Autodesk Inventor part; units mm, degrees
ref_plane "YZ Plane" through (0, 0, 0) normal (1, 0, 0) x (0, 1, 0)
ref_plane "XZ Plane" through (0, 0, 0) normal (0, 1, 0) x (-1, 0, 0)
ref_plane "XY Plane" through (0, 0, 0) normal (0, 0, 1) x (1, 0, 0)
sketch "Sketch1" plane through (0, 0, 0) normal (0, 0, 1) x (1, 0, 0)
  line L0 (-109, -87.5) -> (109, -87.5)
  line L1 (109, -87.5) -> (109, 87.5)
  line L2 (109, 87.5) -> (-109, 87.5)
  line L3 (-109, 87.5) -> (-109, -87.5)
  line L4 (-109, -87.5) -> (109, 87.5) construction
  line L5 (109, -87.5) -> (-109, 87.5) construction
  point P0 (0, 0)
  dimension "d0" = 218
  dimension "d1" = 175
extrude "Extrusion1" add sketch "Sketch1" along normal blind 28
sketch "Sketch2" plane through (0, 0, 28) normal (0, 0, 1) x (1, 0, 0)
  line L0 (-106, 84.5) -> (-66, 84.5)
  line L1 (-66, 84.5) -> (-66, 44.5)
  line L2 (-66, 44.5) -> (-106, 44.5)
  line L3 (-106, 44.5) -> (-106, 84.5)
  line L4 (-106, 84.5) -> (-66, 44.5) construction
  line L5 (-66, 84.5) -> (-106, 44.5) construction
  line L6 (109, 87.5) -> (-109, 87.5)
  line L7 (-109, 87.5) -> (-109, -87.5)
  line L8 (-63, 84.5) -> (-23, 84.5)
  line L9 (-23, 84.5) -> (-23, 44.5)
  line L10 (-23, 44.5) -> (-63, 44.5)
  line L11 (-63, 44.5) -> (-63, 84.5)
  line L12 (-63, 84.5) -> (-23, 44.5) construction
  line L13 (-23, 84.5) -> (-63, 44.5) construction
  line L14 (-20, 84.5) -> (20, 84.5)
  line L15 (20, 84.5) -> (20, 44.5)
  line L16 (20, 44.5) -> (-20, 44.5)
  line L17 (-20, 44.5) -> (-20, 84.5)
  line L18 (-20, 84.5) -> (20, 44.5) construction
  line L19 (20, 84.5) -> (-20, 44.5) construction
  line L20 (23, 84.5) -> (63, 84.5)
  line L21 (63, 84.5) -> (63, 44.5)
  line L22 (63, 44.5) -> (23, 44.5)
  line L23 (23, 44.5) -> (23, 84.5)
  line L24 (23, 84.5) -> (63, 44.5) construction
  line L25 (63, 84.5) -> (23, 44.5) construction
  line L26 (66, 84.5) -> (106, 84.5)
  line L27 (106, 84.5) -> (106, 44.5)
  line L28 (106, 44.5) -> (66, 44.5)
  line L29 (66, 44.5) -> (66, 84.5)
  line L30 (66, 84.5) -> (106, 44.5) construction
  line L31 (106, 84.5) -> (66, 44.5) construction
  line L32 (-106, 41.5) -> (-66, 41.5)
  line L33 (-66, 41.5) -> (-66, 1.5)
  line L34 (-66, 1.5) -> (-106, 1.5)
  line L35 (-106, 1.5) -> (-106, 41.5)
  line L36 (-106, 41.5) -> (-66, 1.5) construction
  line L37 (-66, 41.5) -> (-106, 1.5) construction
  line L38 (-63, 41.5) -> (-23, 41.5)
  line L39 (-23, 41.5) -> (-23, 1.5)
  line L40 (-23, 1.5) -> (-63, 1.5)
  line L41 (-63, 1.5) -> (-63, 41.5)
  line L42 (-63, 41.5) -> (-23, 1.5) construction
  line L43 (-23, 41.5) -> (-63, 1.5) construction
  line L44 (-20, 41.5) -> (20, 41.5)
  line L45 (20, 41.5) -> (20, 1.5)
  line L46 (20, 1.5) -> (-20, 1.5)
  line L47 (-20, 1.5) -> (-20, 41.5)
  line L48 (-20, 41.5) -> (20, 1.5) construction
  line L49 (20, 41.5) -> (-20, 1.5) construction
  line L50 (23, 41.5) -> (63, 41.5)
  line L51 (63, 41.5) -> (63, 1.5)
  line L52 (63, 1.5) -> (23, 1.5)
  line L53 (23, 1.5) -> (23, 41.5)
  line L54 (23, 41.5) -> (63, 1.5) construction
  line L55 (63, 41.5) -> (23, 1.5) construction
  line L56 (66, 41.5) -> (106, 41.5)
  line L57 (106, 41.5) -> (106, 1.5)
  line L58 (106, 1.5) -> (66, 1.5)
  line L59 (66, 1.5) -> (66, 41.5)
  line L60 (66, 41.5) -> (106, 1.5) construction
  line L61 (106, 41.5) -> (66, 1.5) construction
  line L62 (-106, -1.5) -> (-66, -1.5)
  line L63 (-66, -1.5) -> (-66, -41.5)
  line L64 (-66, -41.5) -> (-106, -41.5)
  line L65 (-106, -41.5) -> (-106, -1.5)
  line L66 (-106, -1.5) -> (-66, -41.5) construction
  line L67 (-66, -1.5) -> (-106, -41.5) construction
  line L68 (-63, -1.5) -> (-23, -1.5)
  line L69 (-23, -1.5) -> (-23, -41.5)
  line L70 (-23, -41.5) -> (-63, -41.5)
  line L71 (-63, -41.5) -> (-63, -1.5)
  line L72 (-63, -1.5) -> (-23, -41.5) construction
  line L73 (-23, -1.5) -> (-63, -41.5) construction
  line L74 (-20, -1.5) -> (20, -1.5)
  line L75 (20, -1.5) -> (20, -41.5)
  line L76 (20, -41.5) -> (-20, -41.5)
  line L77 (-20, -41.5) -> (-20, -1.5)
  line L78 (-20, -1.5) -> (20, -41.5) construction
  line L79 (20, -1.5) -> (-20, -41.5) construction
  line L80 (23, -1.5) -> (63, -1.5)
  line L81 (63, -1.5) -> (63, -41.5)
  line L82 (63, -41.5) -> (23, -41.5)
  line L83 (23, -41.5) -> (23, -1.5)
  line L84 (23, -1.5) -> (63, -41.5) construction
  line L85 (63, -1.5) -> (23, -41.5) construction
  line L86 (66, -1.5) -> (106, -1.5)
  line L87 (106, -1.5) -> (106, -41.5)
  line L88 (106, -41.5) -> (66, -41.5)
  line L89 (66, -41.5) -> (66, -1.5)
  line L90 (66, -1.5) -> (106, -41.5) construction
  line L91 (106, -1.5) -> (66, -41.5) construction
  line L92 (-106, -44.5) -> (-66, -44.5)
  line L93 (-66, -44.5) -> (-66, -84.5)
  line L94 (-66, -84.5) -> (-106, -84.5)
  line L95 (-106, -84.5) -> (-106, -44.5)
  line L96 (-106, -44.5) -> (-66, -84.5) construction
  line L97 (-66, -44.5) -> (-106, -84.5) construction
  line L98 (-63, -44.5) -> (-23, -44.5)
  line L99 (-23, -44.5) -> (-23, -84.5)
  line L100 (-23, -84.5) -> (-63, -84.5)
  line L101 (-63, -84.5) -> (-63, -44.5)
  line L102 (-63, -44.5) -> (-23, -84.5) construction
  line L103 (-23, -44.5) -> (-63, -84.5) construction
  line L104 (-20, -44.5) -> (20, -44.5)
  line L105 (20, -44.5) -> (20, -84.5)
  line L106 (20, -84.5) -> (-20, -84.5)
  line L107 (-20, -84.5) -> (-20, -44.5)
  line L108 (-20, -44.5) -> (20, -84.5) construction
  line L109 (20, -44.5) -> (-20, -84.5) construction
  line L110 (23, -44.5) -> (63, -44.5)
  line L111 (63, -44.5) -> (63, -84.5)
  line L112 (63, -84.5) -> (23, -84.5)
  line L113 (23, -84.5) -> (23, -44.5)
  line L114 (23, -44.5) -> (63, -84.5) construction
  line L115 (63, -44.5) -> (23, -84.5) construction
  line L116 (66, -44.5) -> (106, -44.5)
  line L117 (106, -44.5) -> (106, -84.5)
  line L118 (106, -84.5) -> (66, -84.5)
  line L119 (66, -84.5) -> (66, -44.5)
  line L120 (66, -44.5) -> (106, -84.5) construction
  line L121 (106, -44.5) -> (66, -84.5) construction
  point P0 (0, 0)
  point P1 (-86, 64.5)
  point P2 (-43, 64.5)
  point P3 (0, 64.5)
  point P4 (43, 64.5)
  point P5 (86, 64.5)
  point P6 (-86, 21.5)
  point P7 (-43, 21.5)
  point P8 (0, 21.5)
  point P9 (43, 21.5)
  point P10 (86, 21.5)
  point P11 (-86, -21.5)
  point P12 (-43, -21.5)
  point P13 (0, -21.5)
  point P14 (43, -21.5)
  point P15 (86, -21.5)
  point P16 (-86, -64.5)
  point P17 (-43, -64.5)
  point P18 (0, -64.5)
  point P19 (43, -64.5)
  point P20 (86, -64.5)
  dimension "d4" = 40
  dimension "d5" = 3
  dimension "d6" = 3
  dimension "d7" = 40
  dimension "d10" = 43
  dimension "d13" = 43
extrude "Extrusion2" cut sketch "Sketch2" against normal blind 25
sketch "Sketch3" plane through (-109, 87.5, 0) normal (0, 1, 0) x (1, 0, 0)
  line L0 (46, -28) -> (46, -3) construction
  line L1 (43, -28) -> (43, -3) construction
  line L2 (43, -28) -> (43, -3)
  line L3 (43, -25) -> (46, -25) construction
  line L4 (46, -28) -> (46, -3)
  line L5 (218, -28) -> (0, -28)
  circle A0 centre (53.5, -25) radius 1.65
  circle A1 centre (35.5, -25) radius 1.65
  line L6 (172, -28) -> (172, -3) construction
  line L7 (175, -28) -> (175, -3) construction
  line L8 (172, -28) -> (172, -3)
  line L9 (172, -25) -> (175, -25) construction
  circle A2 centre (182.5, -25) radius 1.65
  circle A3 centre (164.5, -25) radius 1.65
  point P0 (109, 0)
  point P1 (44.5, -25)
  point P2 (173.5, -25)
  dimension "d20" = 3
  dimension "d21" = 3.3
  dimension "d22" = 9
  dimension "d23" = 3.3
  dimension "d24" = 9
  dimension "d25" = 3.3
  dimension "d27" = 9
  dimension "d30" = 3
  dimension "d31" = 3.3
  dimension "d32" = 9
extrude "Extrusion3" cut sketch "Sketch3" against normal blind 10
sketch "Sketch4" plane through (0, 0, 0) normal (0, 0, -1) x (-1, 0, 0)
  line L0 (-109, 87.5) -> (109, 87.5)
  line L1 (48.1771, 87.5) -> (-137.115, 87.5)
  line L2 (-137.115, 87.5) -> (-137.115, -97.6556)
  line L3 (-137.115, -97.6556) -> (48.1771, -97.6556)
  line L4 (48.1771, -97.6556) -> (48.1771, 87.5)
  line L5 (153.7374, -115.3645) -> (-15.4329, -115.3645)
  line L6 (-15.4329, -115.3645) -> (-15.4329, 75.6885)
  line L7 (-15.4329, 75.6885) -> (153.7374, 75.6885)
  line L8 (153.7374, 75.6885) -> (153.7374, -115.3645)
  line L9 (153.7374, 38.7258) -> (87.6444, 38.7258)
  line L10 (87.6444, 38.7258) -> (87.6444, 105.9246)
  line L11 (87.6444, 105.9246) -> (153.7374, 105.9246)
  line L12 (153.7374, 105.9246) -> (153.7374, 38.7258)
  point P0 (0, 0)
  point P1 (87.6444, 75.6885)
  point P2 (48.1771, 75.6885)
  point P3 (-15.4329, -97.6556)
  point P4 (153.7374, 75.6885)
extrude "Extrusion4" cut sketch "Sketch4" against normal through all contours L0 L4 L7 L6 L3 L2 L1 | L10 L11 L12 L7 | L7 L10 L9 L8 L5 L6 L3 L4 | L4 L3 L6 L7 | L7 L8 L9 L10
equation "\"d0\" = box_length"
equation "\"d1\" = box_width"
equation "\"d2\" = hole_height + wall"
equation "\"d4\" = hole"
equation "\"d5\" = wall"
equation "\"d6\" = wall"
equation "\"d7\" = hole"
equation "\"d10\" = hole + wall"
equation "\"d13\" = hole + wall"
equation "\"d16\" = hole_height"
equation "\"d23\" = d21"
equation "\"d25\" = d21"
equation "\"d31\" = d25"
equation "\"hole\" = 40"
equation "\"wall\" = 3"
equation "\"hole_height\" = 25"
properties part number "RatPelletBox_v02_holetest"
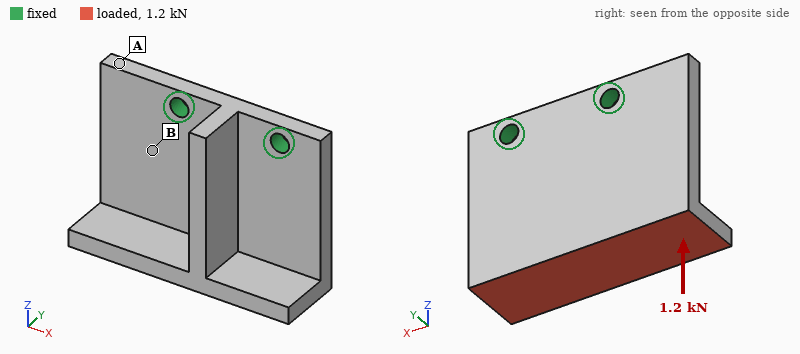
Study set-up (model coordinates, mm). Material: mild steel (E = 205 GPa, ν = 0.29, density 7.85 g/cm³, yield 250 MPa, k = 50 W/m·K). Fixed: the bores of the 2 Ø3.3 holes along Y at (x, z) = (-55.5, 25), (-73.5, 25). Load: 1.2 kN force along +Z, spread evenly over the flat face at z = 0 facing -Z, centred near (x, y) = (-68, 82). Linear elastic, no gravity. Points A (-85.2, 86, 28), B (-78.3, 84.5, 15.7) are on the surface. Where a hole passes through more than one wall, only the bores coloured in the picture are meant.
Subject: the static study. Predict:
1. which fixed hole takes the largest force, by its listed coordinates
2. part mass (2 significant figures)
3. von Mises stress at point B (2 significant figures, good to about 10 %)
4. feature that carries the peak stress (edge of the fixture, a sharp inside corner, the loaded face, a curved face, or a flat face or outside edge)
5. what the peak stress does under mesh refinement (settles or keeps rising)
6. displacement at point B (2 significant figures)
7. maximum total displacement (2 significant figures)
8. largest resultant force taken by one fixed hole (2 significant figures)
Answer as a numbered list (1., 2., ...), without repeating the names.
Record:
1. (-73.5, 25)
2. 39 g
3. 43 MPa
4. edge of the fixture
5. keeps rising
6. 11 µm
7. 67 µm
8. 800 N
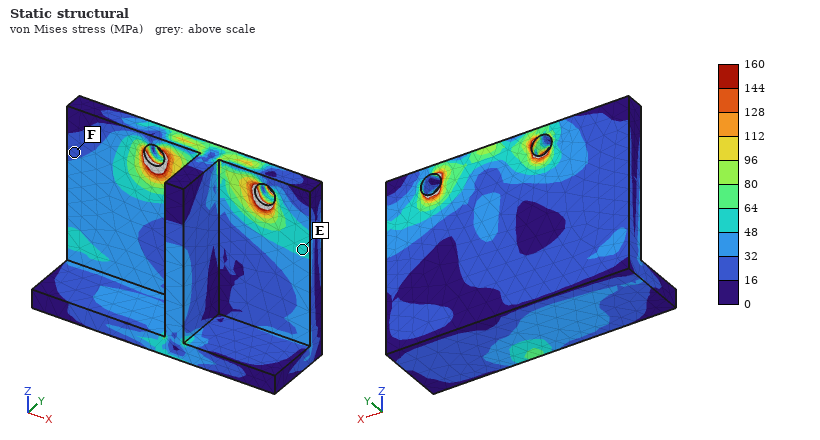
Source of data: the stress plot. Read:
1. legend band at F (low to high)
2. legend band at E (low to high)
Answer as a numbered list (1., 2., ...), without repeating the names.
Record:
1. 16 to 32 MPa
2. 48 to 64 MPa
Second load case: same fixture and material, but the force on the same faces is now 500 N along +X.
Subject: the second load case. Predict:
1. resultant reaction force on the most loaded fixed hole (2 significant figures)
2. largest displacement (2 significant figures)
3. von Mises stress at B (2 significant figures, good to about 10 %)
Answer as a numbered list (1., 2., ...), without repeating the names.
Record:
1. 670 N
2. 22 µm
3. 15 MPa
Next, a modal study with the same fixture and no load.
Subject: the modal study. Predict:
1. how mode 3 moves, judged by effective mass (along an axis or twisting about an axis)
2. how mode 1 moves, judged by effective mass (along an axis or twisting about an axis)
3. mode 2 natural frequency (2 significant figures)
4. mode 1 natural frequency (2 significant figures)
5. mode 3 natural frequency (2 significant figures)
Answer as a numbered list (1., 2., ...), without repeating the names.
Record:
1. along X
2. along Y
3. 4800 Hz
4. 2800 Hz
5. 12 kHz
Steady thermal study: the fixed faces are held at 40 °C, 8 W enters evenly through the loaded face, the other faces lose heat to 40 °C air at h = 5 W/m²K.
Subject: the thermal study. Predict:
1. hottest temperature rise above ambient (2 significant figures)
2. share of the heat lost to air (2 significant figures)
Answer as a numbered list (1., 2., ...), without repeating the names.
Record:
1. 36 K
2. 3.7 %
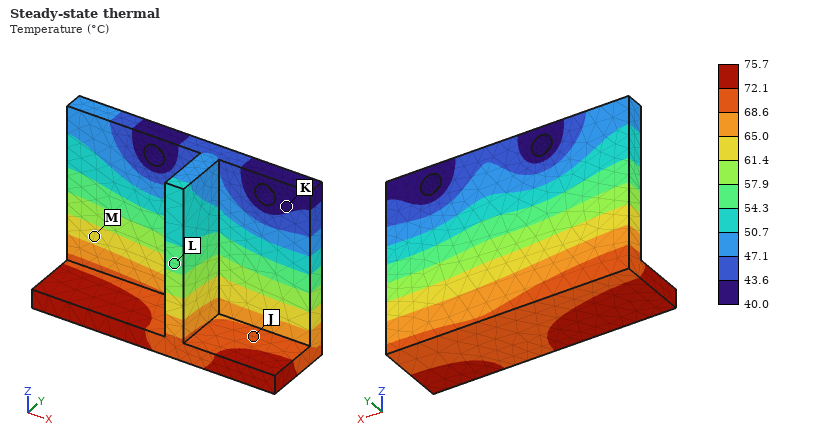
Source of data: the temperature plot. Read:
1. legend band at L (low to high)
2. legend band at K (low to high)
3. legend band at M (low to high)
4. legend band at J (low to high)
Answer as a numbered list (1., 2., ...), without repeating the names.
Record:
1. 54.3 to 57.9 °C
2. 40.0 to 43.6 °C
3. 61.4 to 65.0 °C
4. 68.6 to 72.1 °C
